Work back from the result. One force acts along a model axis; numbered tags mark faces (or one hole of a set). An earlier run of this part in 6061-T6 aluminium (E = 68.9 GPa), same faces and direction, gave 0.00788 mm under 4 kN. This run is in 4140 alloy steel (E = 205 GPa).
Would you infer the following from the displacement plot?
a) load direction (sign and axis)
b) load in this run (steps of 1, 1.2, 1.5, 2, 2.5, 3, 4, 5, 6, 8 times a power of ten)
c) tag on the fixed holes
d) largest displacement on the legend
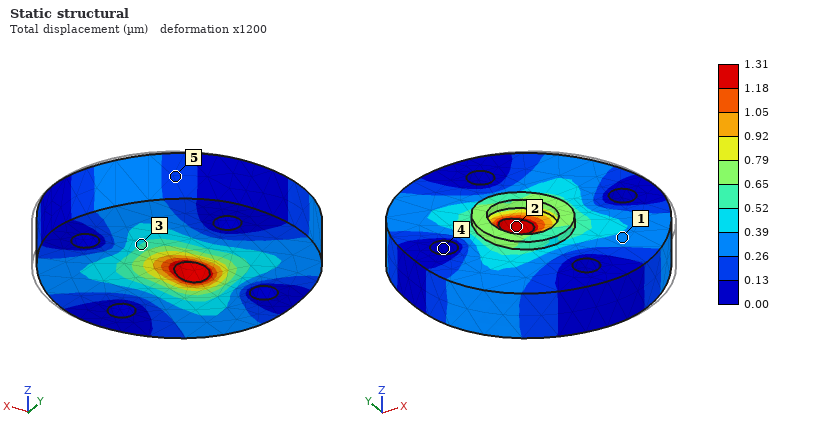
-X
2 kN
4
1.31 µm
